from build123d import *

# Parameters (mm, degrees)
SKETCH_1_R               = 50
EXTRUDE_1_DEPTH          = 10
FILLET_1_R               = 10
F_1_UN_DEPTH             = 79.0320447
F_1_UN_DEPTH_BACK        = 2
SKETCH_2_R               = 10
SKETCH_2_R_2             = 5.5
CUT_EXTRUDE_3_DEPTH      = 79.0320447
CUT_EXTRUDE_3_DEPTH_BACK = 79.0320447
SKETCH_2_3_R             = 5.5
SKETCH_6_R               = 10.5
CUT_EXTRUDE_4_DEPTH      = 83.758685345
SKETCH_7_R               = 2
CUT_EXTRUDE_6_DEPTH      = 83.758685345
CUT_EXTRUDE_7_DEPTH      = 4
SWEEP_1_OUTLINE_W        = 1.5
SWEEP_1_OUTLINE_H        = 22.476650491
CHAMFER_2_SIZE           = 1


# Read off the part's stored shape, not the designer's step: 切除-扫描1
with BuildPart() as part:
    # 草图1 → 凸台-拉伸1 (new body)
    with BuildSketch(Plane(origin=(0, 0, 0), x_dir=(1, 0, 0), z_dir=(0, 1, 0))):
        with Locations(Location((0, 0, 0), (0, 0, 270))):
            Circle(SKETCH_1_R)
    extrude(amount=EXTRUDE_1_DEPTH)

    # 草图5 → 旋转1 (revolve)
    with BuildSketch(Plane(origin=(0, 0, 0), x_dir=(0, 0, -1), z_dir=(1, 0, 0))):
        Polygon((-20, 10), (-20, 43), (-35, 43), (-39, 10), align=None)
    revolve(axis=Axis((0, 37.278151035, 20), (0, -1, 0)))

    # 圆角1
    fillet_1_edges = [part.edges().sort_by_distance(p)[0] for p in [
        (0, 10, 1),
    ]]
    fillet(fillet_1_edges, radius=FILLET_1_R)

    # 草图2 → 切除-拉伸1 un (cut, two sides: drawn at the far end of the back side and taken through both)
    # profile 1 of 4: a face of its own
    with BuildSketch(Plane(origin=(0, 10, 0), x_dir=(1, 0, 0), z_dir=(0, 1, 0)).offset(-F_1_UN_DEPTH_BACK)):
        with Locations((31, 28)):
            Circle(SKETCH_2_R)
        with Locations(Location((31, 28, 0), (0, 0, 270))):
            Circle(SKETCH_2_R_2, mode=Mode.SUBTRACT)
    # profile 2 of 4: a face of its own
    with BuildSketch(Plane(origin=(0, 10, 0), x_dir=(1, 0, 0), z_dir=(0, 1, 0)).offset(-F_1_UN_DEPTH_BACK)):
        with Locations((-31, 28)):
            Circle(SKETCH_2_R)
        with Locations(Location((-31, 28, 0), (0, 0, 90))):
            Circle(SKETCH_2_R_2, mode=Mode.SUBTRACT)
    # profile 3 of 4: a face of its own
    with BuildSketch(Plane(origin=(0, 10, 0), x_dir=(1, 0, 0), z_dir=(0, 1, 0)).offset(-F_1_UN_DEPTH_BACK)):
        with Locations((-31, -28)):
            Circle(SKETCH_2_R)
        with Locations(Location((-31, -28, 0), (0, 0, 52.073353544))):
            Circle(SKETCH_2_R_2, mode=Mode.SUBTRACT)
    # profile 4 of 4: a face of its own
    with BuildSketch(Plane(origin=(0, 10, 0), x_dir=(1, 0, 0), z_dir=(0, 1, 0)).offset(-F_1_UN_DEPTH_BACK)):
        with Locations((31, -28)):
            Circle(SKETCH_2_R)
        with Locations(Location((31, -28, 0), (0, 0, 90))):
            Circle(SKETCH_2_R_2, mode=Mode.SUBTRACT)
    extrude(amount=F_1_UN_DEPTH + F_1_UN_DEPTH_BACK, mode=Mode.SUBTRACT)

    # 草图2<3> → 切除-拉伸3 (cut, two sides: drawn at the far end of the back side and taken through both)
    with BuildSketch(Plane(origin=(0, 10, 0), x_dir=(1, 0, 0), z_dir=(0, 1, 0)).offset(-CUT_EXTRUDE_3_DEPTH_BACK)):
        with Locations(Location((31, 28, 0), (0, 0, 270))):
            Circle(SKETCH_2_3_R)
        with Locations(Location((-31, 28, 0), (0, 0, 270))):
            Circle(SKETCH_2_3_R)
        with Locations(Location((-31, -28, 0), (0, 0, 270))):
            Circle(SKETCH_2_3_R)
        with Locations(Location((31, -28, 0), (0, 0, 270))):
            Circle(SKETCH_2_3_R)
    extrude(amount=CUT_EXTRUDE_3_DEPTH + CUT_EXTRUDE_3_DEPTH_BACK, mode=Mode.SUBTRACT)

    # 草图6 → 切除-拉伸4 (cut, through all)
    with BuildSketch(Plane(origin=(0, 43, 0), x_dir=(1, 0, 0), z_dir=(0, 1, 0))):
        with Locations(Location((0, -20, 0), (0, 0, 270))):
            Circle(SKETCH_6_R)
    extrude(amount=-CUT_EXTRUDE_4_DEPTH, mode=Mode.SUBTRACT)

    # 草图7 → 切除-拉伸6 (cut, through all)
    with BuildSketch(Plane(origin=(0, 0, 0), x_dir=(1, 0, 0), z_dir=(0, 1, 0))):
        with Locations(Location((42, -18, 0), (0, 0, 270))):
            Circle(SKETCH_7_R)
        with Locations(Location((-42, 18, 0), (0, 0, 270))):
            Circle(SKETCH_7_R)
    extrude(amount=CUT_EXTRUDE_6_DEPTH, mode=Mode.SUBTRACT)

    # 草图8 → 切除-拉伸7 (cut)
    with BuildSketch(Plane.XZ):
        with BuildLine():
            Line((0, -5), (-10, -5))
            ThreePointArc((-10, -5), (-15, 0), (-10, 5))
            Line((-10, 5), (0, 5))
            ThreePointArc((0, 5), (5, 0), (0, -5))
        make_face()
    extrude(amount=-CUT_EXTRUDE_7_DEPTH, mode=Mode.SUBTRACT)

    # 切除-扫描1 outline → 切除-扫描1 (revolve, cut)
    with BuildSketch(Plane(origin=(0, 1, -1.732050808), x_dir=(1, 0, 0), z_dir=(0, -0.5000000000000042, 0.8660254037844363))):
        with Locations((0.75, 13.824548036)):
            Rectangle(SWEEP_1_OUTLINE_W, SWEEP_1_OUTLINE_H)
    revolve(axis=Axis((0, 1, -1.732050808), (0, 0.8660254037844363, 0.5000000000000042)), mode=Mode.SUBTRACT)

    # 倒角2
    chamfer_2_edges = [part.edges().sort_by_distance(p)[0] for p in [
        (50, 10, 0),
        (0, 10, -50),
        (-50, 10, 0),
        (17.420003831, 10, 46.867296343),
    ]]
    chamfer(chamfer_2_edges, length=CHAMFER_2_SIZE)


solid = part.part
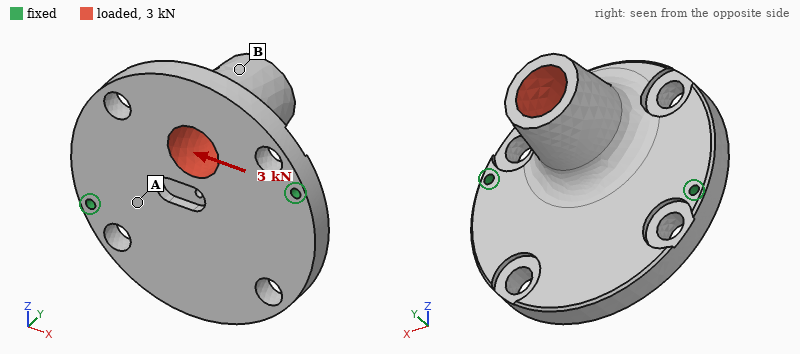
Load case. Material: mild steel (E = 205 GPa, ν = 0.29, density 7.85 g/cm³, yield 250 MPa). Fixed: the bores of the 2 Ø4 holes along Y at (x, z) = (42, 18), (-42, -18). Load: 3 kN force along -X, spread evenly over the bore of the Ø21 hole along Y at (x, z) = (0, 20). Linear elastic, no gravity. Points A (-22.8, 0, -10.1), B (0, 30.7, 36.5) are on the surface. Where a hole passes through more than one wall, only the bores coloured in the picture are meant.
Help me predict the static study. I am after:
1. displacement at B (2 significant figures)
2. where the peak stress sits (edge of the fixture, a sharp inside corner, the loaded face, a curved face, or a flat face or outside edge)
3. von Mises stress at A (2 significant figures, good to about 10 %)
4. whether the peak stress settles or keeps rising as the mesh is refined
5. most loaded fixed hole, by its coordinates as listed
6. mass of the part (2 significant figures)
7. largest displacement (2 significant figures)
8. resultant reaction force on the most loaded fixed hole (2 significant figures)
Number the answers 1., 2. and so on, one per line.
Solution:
1. 21 µm
2. edge of the fixture
3. 11 MPa
4. keeps rising
5. (42, 18)
6. 700 g
7. 27 µm
8. 1.9 kN
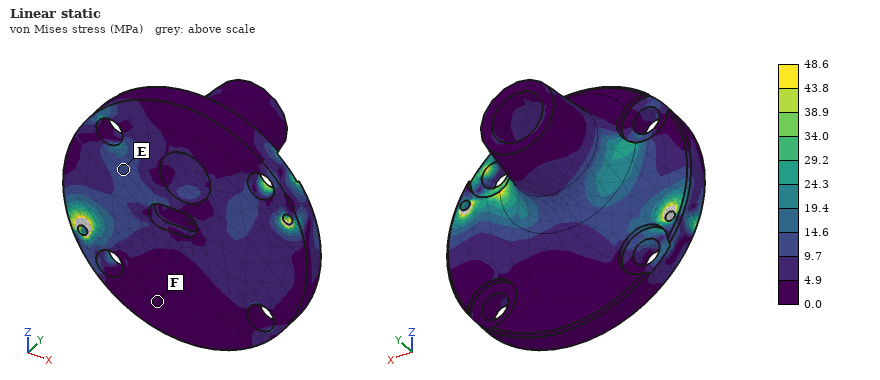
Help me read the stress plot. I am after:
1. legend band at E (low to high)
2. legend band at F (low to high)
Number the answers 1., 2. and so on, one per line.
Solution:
1. 9.7 to 14.6 MPa
2. 0.0 to 4.9 MPa
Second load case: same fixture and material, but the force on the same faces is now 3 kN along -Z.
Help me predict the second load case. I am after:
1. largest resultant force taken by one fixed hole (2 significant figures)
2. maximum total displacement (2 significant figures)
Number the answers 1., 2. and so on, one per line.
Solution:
1. 1.6 kN
2. 57 µm
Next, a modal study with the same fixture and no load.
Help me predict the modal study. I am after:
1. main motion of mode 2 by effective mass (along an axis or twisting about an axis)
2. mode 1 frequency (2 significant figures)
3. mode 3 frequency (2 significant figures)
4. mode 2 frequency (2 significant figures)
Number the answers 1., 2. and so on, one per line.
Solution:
1. along Y
2. 1600 Hz
3. 5800 Hz
4. 2900 Hz
